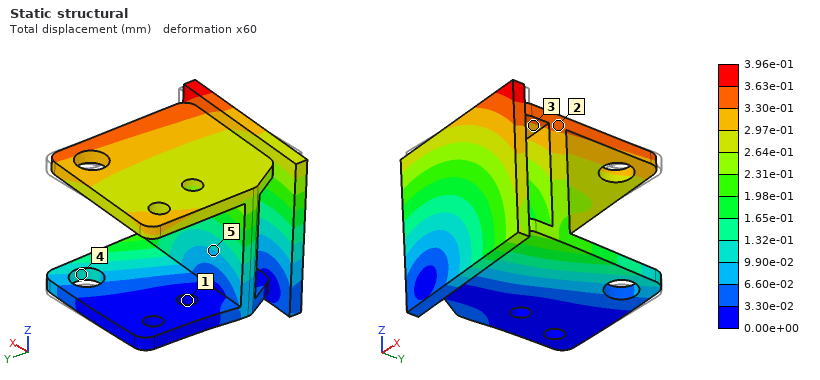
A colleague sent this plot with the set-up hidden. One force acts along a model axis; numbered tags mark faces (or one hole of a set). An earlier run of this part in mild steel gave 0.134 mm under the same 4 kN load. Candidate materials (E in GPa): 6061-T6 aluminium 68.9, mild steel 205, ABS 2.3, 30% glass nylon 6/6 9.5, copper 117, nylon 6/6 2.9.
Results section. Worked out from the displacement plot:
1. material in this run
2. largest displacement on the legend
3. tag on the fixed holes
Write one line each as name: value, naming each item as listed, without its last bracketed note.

material in this run: 6061-T6 aluminium
largest displacement on the legend: 3.96e-01 mm
tag on the fixed holes: 1
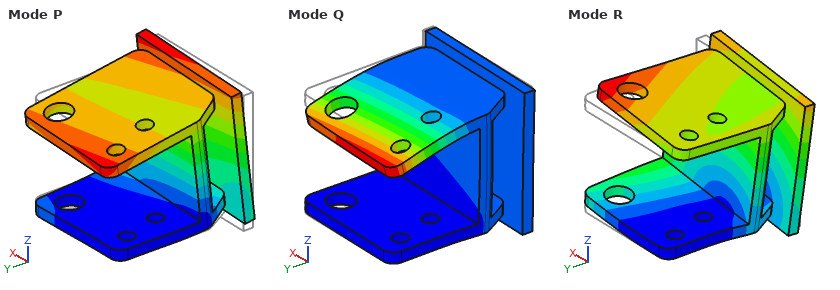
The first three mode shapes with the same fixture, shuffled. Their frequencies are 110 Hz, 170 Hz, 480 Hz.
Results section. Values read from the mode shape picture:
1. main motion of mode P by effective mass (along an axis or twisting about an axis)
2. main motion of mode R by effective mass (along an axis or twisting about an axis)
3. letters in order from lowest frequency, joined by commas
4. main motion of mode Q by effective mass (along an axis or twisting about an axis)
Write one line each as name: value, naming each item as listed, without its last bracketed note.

main motion of mode P by effective mass: along Y
main motion of mode R by effective mass: along X
letters in order from lowest frequency, joined by commas: P, R, Q
main motion of mode Q by effective mass: along Z
